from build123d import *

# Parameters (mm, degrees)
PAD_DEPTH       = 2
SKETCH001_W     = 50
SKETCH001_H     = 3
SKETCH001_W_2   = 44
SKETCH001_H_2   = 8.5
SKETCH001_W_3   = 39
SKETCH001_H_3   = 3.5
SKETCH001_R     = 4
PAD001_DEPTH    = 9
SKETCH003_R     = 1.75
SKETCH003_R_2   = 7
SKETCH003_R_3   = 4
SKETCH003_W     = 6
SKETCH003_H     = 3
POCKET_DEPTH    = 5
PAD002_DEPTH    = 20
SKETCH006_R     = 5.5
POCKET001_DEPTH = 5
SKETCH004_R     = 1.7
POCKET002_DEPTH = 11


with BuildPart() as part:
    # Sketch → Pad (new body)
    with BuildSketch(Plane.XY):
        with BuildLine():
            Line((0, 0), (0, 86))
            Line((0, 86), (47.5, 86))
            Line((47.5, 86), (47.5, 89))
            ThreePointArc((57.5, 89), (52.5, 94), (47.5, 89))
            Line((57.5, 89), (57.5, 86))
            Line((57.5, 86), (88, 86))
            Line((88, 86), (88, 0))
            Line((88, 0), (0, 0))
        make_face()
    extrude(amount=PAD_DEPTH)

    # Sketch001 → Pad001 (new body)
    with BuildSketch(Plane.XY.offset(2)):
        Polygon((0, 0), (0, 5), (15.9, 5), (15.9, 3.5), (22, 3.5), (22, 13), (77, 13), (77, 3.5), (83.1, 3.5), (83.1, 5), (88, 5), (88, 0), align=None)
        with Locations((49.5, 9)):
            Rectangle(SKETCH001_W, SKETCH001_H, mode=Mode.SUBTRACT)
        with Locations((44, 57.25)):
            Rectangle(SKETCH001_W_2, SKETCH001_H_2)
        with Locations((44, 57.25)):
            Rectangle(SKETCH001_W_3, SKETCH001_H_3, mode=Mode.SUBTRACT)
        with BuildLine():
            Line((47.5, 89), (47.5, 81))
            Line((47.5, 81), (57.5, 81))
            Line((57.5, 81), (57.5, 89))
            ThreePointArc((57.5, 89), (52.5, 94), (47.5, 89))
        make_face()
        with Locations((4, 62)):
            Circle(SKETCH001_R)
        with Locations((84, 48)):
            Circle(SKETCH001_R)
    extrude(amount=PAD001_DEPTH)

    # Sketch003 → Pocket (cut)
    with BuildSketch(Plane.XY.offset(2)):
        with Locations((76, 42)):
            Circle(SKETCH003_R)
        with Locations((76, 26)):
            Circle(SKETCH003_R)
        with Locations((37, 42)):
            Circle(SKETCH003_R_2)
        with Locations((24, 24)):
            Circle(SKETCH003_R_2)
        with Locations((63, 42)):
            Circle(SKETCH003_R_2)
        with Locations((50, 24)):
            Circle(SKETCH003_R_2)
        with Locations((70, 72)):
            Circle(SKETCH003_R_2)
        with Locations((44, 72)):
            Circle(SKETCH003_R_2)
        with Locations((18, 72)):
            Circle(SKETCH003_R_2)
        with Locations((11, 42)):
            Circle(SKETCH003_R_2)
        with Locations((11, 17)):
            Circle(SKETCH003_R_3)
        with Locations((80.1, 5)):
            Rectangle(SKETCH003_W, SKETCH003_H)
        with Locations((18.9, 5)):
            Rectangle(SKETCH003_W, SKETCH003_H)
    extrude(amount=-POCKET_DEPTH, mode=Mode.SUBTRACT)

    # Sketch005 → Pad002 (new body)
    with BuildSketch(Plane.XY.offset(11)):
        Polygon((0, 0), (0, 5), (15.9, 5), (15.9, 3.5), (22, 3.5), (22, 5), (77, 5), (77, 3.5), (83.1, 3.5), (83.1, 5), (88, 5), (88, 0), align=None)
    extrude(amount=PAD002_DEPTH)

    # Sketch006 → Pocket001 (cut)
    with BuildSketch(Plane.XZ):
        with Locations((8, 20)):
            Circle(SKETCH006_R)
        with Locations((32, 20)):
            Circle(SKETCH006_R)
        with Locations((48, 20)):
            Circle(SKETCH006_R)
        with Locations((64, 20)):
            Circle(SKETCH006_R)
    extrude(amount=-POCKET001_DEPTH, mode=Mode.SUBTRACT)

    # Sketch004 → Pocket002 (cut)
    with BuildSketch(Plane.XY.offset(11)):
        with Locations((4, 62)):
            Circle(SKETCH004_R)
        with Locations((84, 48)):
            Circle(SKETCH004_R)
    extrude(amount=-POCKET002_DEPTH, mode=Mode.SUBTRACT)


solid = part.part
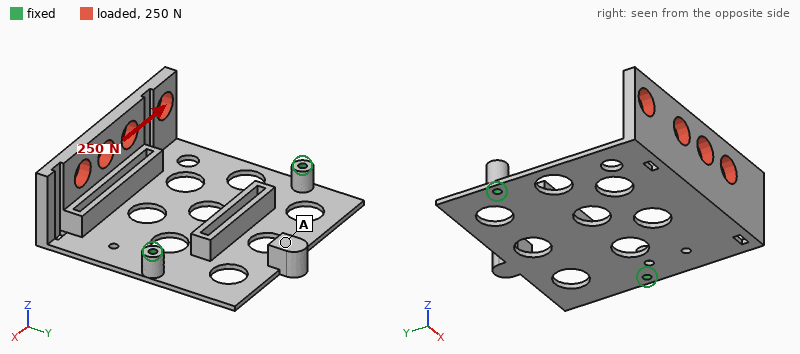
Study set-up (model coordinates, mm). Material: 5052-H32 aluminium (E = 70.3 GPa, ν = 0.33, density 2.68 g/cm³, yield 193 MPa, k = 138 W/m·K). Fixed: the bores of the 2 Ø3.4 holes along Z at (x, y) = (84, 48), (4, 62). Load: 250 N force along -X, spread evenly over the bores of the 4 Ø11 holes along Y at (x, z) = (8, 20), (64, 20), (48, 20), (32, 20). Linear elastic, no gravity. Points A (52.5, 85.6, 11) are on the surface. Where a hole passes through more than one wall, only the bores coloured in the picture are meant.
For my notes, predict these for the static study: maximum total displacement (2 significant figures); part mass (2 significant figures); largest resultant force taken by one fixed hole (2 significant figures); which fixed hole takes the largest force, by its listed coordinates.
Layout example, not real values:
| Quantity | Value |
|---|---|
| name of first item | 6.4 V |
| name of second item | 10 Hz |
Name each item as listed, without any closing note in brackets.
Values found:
| Quantity | Value |
|---|---|
| maximum total displacement | 1.1 mm |
| part mass | 79 g |
| largest resultant force taken by one fixed hole | 220 N |
| which fixed hole takes the largest force, by its listed coordinates | (84, 48) |
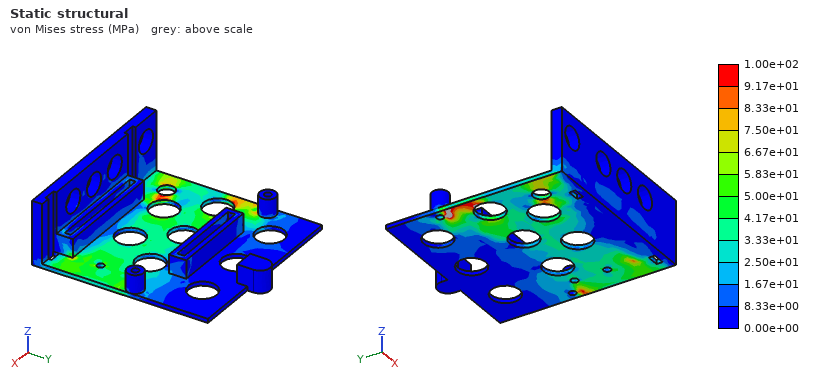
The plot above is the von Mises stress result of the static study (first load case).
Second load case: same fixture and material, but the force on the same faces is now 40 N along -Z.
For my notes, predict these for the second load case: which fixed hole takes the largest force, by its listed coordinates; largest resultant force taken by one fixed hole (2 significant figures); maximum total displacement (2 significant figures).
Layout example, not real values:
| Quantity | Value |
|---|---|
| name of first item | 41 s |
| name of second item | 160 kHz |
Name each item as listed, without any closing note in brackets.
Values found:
| Quantity | Value |
|---|---|
| which fixed hole takes the largest force, by its listed coordinates | (84, 48) |
| largest resultant force taken by one fixed hole | 22 N |
| maximum total displacement | 1.1 mm |
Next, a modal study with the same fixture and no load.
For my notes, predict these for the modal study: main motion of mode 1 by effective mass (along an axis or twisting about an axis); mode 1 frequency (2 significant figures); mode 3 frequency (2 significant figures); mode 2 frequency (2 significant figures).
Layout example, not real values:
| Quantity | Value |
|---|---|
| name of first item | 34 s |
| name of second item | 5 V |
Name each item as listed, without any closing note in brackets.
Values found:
| Quantity | Value |
|---|---|
| main motion of mode 1 by effective mass | along Z |
| mode 1 frequency | 170 Hz |
| mode 3 frequency | 790 Hz |
| mode 2 frequency | 520 Hz |
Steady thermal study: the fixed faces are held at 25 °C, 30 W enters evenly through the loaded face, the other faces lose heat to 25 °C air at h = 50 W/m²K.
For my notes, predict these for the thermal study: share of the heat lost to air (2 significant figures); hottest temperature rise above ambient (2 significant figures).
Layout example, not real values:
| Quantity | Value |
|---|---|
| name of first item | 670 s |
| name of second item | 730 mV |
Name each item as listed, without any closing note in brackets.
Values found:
| Quantity | Value |
|---|---|
| share of the heat lost to air | 76 % |
| hottest temperature rise above ambient | 49 K |
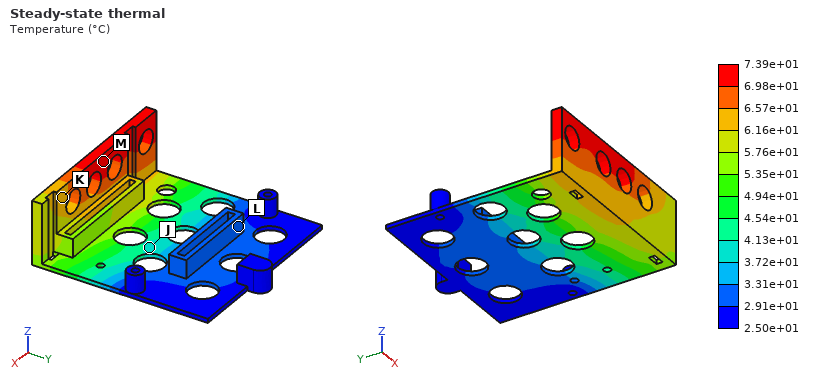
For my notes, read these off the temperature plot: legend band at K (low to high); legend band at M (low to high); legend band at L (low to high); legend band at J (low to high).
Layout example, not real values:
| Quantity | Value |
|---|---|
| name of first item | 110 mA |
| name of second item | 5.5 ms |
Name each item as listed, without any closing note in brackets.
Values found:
| Quantity | Value |
|---|---|
| legend band at K | 6.16e+01 to 6.57e+01 °C |
| legend band at M | 6.98e+01 to 7.39e+01 °C |
| legend band at L | 2.91e+01 to 3.31e+01 °C |
| legend band at J | 3.72e+01 to 4.13e+01 °C |
